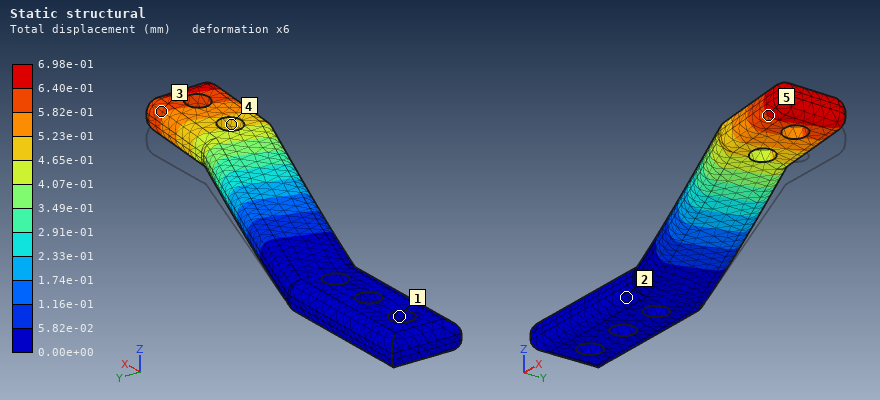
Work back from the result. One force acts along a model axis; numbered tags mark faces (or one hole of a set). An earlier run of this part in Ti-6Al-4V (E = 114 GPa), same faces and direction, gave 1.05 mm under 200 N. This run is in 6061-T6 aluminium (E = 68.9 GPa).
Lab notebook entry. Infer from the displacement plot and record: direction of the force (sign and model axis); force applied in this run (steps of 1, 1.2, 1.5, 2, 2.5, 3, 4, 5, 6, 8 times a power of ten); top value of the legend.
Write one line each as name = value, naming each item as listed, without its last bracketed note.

direction of the force = +Z
force applied in this run = 80 N
top value of the legend = 6.98e-01 mm
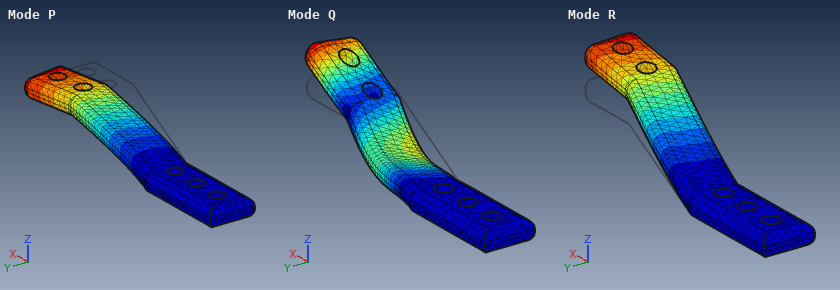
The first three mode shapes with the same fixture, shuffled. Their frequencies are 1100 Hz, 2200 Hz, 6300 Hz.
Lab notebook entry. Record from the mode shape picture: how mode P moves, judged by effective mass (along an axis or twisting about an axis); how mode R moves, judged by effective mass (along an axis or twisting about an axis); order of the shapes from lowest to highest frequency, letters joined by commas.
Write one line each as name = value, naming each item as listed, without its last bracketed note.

how mode P moves, judged by effective mass = along Y
how mode R moves, judged by effective mass = along Z
order of the shapes from lowest to highest frequency, letters joined by commas = R, P, Q
